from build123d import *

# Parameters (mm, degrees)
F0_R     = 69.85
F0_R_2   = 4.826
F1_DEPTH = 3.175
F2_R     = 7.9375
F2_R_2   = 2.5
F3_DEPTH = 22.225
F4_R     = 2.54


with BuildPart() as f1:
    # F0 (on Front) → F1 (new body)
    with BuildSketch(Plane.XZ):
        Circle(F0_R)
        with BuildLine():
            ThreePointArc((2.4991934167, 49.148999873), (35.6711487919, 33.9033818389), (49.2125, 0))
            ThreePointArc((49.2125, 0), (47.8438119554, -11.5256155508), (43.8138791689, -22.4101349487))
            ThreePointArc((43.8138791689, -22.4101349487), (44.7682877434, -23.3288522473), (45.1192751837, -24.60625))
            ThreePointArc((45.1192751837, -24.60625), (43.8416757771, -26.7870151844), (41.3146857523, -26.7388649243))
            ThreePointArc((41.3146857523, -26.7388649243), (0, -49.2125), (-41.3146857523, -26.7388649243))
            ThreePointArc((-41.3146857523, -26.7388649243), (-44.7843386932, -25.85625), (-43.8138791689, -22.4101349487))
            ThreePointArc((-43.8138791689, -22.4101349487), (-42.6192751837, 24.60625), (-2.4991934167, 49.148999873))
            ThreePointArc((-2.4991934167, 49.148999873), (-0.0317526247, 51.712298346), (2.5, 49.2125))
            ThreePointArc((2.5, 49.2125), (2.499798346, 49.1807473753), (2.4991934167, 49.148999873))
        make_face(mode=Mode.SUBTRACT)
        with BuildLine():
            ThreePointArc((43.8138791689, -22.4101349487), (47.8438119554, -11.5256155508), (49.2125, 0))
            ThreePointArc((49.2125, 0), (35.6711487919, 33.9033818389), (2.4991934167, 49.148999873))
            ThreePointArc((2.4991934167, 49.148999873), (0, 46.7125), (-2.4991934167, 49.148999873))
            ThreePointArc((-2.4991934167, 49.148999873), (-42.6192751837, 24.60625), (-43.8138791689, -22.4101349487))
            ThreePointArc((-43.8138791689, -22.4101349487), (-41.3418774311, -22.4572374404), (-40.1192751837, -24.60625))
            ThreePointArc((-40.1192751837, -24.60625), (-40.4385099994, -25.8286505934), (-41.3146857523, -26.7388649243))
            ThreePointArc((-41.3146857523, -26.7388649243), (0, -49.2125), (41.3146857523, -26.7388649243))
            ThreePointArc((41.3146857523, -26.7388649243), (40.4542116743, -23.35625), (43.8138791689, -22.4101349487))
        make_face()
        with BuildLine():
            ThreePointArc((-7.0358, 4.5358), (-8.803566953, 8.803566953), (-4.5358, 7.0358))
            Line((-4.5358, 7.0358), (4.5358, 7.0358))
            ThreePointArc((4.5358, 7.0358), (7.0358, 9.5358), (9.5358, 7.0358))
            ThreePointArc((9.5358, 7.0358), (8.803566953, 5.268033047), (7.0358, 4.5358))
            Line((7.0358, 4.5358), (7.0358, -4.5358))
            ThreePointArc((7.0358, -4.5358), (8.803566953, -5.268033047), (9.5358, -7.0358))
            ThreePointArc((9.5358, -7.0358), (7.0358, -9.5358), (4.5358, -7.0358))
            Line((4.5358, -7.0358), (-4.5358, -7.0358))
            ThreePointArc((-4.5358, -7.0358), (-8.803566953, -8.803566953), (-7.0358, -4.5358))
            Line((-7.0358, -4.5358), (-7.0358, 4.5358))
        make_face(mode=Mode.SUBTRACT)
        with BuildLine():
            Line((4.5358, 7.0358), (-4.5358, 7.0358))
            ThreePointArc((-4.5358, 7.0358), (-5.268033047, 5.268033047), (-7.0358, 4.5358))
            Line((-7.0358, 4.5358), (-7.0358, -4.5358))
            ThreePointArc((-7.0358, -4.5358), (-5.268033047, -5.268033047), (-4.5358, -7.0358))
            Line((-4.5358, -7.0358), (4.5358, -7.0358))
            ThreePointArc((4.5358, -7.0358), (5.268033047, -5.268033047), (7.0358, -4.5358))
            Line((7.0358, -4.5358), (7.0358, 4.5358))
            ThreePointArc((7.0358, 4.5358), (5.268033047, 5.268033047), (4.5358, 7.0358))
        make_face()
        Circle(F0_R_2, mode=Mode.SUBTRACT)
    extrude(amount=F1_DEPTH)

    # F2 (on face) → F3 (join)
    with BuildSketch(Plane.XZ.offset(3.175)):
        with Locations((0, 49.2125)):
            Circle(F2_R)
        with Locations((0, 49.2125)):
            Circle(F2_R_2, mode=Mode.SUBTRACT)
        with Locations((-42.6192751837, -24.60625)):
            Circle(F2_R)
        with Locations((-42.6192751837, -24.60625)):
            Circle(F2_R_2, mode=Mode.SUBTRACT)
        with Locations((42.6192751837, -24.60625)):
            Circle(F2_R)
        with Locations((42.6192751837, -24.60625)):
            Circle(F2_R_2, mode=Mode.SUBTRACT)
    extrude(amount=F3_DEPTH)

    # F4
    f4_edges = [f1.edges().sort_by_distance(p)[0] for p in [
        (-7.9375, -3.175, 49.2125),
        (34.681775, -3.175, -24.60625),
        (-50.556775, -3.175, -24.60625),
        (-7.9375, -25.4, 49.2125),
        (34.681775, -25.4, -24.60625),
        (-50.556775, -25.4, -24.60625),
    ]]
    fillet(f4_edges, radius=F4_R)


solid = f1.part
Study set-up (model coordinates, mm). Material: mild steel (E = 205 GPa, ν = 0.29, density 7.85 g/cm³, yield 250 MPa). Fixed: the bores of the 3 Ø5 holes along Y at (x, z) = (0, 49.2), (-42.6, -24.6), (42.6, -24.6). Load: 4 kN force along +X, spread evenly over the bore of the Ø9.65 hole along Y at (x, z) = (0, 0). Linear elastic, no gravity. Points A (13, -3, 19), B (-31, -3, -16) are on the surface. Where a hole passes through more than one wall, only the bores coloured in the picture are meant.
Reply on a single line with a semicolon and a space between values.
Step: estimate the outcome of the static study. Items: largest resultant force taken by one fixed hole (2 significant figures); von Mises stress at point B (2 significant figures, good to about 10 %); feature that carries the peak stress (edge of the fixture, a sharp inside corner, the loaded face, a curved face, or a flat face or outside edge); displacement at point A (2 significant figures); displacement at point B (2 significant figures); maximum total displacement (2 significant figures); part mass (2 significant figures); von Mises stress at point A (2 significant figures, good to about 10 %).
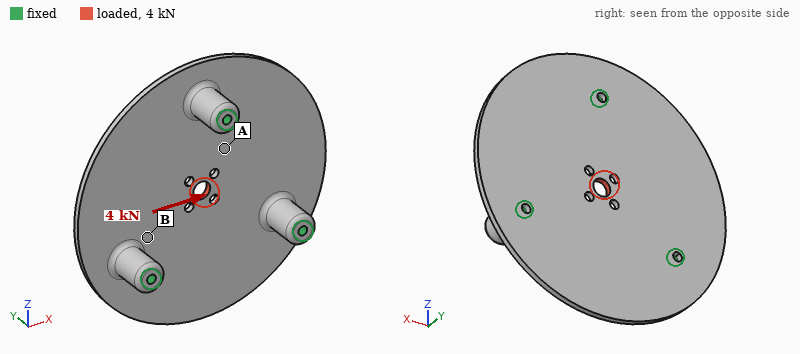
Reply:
1.4 kN; 20 MPa; a curved face; 2.9 µm; 1.9 µm; 6.7 µm; 470 g; 10.0 MPa
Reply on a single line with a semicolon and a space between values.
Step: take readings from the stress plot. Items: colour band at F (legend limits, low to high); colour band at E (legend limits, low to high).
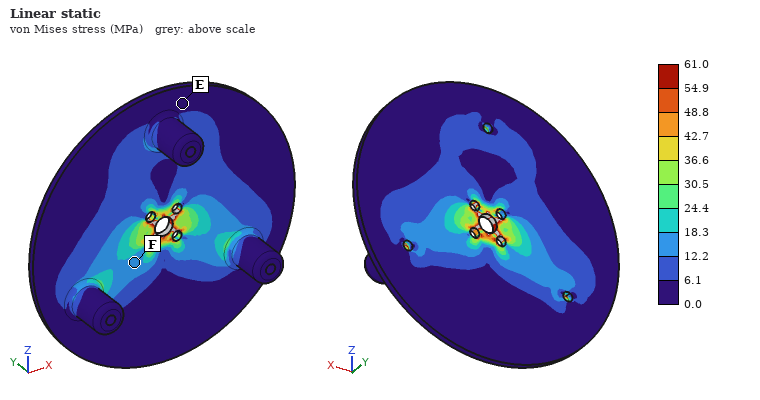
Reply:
12.2 to 18.3 MPa; 0.0 to 6.1 MPa
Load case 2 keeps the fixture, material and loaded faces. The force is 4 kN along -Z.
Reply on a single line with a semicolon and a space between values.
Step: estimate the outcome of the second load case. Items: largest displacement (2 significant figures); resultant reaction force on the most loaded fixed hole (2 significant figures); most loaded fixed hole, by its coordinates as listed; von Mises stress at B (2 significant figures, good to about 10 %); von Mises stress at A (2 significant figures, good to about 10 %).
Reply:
6.6 µm; 1.5 kN; (0, 49.2); 13 MPa; 13 MPa
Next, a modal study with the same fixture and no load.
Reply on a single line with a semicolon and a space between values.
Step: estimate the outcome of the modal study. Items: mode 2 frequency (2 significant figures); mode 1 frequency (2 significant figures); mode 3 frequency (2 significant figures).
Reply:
1500 Hz; 1500 Hz; 1500 Hz
